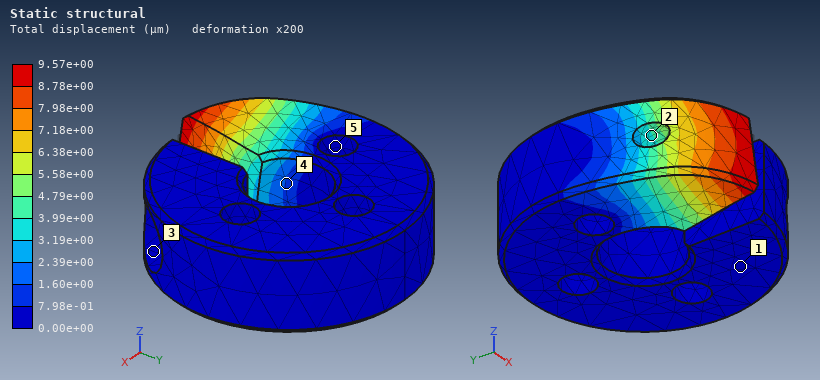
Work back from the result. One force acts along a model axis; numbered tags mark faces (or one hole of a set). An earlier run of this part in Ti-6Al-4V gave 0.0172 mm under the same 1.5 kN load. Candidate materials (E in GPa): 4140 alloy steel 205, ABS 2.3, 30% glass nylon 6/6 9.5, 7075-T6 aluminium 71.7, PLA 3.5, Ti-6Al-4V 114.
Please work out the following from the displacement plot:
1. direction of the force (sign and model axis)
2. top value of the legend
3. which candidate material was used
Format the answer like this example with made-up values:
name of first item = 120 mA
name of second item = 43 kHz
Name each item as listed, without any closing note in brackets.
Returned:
direction of the force = +Z
top value of the legend = 9.57e+00 µm
which candidate material was used = 4140 alloy steel
